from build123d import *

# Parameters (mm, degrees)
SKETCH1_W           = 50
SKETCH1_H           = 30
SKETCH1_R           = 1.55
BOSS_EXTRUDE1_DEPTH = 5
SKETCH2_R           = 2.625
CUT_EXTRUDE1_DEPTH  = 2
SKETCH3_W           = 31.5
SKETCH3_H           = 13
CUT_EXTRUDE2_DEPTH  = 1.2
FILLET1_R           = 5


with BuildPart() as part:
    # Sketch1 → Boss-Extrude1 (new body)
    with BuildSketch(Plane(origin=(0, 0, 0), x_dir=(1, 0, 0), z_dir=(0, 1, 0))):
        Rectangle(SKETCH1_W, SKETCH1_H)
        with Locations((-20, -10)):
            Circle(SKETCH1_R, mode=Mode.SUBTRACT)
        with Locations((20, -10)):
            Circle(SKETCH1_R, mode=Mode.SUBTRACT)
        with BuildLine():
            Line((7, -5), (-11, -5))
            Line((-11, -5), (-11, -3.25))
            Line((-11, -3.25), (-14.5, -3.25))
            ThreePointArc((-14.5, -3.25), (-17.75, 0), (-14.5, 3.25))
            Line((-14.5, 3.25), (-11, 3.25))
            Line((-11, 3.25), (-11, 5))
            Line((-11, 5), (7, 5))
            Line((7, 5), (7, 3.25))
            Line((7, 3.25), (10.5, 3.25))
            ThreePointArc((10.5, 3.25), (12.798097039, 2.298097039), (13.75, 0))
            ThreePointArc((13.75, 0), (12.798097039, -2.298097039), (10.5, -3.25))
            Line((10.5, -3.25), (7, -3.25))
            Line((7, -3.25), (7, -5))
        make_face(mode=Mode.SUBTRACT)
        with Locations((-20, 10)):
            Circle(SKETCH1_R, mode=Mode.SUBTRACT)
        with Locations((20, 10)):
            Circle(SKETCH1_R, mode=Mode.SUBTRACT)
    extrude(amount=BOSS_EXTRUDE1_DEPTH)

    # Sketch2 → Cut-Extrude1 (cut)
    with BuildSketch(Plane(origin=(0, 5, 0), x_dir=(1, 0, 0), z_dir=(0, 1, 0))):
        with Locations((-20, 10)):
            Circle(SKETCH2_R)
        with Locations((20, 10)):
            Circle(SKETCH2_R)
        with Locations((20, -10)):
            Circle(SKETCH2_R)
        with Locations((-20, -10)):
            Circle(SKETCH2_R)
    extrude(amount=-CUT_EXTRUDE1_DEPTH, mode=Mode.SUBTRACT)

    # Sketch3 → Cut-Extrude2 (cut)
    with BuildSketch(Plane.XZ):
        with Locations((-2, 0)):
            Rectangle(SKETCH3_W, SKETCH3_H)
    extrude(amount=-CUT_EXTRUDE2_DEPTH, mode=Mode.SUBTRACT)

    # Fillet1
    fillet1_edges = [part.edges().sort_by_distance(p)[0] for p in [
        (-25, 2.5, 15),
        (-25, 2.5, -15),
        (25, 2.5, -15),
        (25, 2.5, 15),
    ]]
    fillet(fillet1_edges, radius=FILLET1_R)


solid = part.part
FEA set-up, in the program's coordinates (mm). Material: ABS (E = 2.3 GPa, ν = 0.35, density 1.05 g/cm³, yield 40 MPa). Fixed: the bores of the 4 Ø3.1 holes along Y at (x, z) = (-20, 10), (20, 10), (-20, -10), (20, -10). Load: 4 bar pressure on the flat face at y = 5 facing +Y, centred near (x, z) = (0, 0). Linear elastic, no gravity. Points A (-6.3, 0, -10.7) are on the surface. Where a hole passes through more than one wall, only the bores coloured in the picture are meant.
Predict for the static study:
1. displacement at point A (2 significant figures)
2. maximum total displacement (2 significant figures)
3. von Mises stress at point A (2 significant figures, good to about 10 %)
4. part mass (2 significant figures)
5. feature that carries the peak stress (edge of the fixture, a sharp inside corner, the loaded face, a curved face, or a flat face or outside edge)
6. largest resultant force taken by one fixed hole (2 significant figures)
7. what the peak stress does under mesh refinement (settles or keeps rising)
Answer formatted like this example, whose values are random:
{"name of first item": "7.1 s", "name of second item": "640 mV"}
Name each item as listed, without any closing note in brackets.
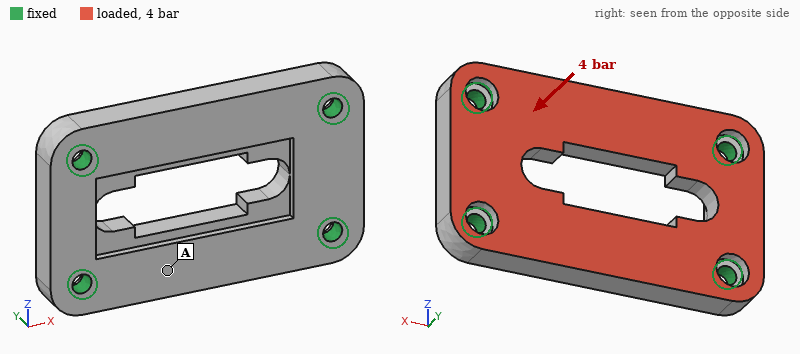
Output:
{"displacement at point A": "0.15 mm", "maximum total displacement": "0.19 mm", "von Mises stress at point A": "5.0 MPa", "part mass": "5.9 g", "feature that carries the peak stress": "edge of the fixture", "largest resultant force taken by one fixed hole": "130 N", "what the peak stress does under mesh refinement": "keeps rising"}
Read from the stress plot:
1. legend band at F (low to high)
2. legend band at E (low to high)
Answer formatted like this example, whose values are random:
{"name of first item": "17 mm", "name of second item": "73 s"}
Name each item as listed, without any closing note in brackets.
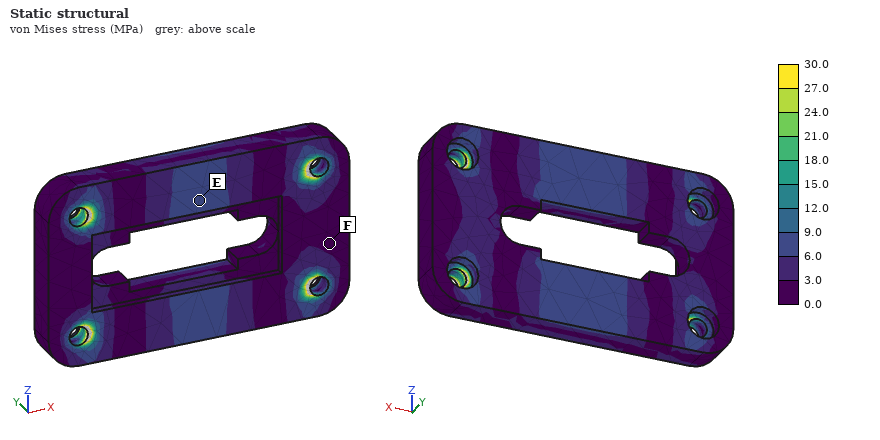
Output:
{"legend band at F": "0.0 to 3.0 MPa", "legend band at E": "6.0 to 9.0 MPa"}
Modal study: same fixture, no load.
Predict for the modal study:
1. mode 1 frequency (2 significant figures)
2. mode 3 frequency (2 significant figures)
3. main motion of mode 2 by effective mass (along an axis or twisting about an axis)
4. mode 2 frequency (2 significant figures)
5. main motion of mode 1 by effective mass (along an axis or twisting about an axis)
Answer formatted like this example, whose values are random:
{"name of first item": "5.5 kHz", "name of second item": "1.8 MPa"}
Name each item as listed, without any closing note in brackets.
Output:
{"mode 1 frequency": "3700 Hz", "mode 3 frequency": "6700 Hz", "main motion of mode 2 by effective mass": "twisting about X", "mode 2 frequency": "4100 Hz", "main motion of mode 1 by effective mass": "along Y"}
